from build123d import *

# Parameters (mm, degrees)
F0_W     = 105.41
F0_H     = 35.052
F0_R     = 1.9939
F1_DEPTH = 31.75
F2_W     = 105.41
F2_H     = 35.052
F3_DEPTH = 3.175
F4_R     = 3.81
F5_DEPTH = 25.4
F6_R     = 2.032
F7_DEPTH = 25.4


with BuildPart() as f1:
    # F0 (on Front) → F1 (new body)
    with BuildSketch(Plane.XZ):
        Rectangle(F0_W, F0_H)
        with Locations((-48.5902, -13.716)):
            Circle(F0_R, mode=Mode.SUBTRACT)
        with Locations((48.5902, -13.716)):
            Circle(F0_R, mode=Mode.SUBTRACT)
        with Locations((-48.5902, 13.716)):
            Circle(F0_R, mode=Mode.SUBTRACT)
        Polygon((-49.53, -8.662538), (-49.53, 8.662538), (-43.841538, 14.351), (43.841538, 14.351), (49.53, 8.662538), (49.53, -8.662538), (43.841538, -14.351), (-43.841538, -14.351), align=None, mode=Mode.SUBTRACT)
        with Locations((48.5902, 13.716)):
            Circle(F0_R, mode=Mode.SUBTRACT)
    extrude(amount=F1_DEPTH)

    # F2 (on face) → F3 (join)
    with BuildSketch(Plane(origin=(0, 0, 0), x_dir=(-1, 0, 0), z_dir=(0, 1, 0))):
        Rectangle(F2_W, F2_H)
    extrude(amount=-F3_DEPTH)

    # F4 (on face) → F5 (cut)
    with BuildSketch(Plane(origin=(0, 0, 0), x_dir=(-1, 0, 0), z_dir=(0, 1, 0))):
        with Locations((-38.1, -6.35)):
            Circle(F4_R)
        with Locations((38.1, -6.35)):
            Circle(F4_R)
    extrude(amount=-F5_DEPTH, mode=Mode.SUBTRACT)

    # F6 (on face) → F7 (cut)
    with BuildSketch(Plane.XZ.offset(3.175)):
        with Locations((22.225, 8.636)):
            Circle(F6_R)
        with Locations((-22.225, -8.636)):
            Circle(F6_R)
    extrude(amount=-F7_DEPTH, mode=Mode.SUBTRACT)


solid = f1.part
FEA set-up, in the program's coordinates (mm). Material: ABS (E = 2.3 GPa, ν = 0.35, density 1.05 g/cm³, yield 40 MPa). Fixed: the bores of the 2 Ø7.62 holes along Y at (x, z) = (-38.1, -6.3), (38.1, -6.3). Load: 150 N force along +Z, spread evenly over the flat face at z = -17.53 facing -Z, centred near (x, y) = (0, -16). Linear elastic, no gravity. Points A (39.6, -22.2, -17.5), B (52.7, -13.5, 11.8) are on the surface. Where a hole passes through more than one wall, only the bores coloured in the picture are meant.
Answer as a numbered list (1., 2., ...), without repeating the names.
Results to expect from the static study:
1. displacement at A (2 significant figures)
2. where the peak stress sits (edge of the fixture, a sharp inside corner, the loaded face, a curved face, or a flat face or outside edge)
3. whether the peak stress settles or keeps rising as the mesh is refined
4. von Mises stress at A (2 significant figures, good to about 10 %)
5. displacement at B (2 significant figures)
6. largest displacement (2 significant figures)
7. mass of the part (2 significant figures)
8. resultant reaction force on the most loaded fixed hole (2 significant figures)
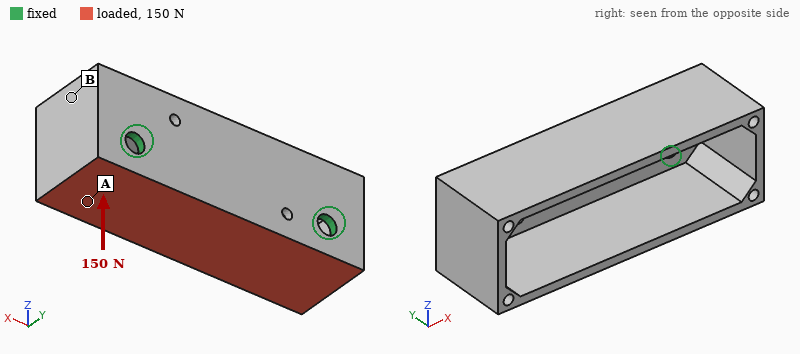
1. 0.32 mm
2. edge of the fixture
3. keeps rising
4. 3.2 MPa
5. 0.23 mm
6. 0.97 mm
7. 38 g
8. 75 N
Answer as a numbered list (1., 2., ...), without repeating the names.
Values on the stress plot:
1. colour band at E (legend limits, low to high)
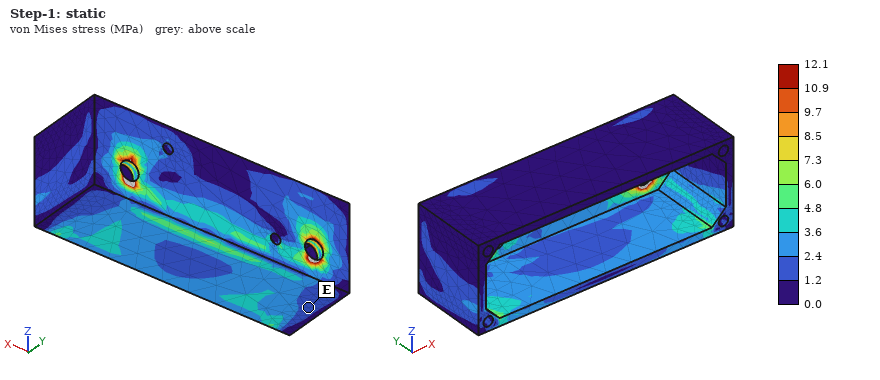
1. 1.2 to 2.4 MPa
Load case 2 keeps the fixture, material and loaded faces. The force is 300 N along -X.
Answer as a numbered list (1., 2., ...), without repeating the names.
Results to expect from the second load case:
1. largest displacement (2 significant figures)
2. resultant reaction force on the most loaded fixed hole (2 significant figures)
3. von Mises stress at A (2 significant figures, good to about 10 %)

1. 0.11 mm
2. 170 N
3. 0.88 MPa
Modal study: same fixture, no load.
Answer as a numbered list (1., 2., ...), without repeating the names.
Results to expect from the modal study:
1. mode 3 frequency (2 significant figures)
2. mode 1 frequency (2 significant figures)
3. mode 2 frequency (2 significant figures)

1. 890 Hz
2. 510 Hz
3. 700 Hz
